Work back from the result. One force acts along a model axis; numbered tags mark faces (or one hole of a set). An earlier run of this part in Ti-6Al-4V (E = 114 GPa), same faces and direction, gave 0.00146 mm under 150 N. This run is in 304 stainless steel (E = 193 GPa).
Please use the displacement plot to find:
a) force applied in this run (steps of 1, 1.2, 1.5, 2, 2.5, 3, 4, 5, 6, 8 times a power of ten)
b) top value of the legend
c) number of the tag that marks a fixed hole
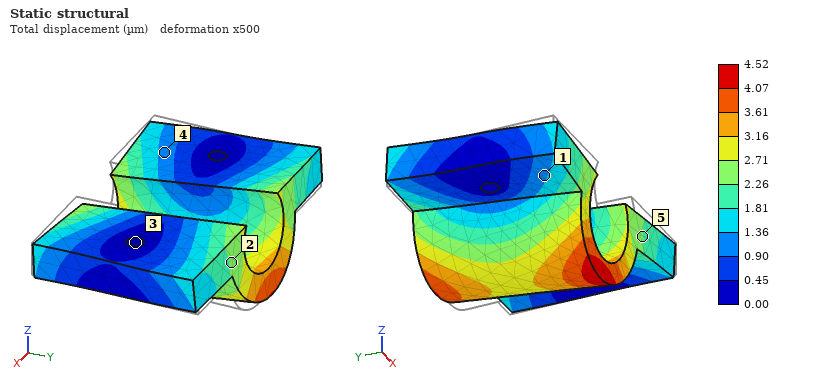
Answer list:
800 N
4.52 µm
3
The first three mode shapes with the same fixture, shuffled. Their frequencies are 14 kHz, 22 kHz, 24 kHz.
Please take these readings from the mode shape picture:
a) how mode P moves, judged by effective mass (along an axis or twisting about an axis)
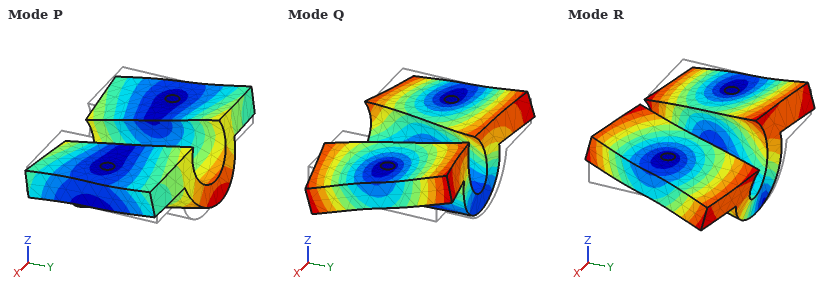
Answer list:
along Y
